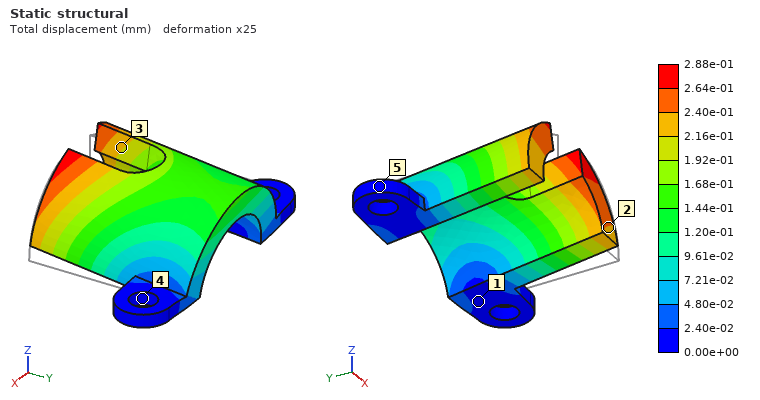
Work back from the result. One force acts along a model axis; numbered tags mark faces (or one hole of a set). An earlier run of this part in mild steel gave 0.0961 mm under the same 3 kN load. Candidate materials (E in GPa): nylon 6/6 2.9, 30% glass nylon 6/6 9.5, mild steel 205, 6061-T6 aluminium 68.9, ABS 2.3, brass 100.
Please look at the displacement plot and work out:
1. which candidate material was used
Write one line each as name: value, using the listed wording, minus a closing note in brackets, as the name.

which candidate material was used: 6061-T6 aluminium
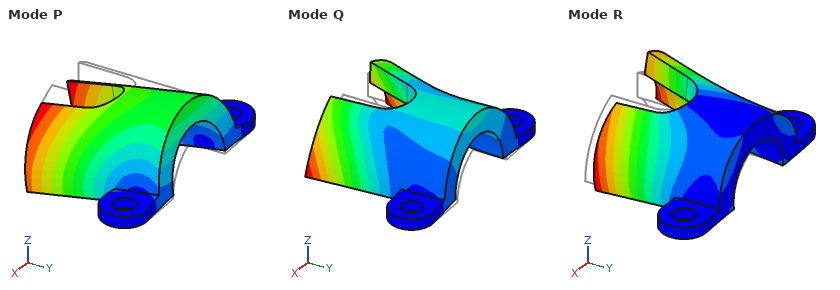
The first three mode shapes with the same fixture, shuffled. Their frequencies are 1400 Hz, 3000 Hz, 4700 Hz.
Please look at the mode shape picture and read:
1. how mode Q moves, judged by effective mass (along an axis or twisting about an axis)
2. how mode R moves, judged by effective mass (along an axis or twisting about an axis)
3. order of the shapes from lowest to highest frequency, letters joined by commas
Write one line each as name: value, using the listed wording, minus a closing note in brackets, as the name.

how mode Q moves, judged by effective mass: along Y
how mode R moves, judged by effective mass: along X
order of the shapes from lowest to highest frequency, letters joined by commas: P, R, Q
